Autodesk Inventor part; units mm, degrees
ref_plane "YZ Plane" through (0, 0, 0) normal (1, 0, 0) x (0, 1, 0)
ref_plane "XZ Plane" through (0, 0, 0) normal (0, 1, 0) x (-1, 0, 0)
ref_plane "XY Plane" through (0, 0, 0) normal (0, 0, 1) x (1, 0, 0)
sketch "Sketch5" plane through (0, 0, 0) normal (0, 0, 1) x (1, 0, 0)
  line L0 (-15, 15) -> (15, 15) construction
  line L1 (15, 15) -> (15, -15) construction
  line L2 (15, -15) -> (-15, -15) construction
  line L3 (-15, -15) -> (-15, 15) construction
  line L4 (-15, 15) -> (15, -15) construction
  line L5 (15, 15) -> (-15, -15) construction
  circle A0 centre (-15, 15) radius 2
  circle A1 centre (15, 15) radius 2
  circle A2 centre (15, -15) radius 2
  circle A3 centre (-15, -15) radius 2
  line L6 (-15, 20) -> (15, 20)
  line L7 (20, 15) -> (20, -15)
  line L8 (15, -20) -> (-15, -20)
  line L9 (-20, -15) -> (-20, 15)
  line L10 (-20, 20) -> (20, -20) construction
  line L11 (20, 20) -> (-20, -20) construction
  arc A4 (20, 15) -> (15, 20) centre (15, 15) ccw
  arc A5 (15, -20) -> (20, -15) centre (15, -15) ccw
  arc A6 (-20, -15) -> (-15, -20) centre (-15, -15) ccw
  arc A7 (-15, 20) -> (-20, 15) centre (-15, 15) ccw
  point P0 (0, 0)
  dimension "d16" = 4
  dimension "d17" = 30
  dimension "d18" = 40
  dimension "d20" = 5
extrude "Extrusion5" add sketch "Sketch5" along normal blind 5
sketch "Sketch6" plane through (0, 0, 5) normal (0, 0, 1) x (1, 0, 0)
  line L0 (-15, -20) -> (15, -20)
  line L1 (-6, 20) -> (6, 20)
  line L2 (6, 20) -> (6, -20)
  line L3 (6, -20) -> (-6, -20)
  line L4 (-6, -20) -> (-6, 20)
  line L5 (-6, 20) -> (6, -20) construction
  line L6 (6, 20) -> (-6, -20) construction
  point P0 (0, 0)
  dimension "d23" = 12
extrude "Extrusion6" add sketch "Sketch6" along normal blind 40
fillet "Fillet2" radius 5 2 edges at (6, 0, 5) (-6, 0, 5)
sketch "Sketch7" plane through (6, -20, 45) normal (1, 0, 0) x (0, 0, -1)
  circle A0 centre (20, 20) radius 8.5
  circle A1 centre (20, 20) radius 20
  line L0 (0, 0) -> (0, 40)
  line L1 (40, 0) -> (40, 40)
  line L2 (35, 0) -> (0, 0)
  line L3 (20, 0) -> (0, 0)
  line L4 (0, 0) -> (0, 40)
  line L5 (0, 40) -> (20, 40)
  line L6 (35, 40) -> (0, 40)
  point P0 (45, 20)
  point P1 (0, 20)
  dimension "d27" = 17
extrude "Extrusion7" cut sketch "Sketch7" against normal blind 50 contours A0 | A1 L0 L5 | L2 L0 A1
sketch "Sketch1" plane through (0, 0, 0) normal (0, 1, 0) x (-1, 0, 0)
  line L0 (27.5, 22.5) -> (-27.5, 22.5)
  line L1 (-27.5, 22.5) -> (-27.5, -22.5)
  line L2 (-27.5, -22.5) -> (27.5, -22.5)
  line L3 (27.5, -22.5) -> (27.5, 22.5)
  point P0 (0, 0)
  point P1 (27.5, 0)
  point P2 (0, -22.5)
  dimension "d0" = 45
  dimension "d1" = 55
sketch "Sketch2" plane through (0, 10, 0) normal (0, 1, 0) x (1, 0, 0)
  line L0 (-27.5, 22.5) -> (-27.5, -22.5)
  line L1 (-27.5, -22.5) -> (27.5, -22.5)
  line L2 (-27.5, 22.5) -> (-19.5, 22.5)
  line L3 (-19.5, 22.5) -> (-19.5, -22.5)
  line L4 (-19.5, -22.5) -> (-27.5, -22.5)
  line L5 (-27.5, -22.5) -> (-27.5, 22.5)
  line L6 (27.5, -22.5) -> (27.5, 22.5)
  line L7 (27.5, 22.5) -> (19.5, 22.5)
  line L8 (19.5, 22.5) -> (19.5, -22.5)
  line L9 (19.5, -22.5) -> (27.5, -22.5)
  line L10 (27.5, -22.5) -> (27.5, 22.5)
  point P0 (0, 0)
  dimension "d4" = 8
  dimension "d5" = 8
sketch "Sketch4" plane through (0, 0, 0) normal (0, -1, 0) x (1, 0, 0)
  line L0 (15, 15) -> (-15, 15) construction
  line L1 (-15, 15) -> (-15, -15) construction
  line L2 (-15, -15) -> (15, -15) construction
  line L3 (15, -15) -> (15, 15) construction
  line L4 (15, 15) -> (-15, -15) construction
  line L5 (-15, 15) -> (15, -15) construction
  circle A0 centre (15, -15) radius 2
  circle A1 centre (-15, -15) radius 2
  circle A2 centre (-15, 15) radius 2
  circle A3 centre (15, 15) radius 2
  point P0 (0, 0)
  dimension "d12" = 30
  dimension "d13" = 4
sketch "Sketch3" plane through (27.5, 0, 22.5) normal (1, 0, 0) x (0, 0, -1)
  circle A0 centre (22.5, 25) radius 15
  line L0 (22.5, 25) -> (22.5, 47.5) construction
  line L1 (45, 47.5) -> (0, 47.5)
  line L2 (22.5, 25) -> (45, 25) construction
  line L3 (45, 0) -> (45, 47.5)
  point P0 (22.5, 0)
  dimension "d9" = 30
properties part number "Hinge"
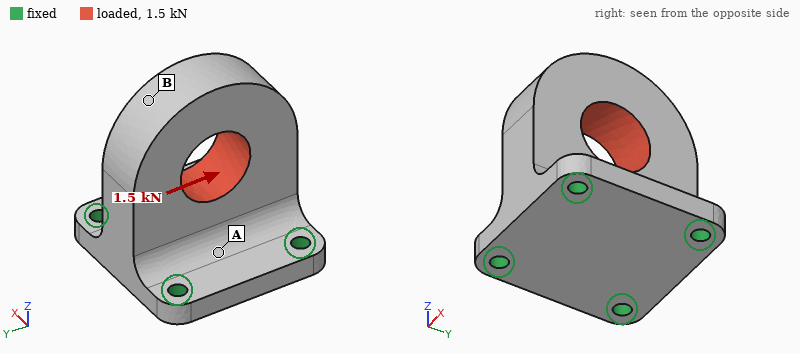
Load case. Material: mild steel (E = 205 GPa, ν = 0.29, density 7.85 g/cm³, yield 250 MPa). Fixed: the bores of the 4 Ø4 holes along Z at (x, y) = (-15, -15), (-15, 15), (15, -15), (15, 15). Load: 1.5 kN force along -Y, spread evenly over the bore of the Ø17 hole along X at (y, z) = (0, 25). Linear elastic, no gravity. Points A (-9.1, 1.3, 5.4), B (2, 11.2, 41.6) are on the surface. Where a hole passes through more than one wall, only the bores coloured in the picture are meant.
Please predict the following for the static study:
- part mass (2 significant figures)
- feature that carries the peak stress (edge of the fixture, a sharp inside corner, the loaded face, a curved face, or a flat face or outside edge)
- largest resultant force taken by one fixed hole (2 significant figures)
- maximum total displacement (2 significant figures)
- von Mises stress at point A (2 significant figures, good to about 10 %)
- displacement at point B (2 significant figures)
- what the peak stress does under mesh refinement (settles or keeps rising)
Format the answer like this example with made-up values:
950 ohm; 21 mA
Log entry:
180 g; edge of the fixture; 760 N; 9.4 µm; 16 MPa; 9.1 µm; keeps rising
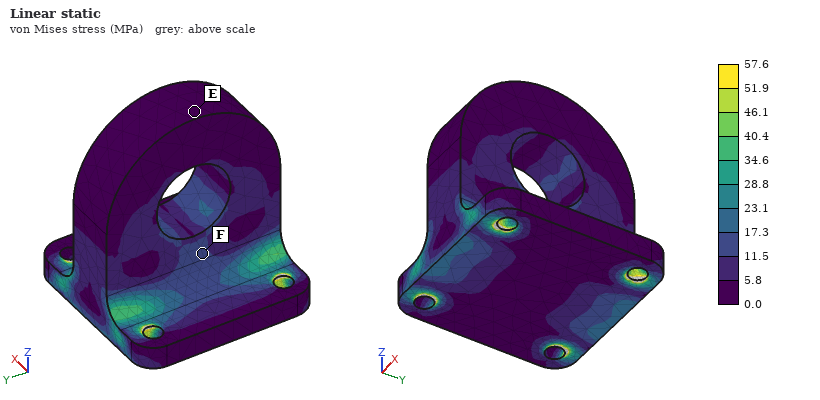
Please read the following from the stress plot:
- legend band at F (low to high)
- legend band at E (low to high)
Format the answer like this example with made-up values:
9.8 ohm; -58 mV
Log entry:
11.5 to 17.3 MPa; 0.0 to 5.8 MPa
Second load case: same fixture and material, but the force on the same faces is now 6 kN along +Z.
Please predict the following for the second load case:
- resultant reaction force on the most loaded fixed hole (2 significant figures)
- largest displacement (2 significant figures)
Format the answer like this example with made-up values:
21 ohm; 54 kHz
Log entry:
1.6 kN; 8.5 µm
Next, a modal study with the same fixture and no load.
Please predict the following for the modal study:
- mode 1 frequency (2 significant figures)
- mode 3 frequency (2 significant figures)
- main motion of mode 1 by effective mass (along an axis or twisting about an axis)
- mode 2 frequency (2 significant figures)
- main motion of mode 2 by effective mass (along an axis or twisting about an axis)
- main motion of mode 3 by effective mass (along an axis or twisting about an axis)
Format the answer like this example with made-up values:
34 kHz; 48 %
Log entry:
5300 Hz; 13 kHz; along X; 7100 Hz; along Y; along Z
